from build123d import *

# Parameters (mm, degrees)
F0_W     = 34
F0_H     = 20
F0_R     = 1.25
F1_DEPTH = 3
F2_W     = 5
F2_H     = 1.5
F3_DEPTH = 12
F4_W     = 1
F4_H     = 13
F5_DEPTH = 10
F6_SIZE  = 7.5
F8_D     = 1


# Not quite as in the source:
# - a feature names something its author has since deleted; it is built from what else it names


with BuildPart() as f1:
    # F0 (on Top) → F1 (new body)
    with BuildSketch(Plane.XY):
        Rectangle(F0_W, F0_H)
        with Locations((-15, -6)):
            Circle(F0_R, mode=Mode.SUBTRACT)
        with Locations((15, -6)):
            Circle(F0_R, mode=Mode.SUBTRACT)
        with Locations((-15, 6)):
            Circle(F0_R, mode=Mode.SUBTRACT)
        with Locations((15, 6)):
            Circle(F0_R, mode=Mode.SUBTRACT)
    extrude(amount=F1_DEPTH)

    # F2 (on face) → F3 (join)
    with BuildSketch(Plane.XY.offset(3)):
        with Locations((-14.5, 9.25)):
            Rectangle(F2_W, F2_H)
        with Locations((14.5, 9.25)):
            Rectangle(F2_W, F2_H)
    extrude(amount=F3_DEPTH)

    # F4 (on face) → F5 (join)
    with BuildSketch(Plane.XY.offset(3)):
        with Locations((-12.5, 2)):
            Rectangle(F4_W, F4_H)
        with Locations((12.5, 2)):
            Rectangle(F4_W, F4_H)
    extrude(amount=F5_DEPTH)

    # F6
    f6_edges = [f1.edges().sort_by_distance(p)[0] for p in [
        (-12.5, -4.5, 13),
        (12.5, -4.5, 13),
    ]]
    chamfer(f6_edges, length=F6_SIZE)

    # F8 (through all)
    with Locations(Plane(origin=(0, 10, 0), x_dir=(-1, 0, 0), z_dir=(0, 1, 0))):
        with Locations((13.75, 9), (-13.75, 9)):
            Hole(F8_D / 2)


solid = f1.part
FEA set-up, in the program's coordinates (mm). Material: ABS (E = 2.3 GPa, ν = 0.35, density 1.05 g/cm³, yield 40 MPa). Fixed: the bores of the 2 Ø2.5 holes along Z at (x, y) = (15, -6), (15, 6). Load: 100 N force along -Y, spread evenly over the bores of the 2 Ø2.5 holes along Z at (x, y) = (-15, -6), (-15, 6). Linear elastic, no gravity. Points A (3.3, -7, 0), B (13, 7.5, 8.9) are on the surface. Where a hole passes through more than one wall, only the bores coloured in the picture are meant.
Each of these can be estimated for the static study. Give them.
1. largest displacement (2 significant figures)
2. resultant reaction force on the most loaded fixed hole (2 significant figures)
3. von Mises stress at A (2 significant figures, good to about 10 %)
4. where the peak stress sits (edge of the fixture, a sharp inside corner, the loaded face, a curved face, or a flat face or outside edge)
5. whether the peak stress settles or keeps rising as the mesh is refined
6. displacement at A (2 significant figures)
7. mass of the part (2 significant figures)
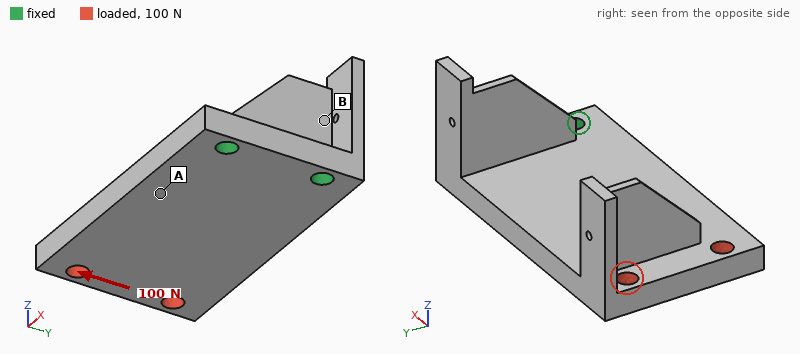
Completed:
0.34 mm
230 N
6.8 MPa
edge of the fixture
keeps rising
0.093 mm
2.5 g
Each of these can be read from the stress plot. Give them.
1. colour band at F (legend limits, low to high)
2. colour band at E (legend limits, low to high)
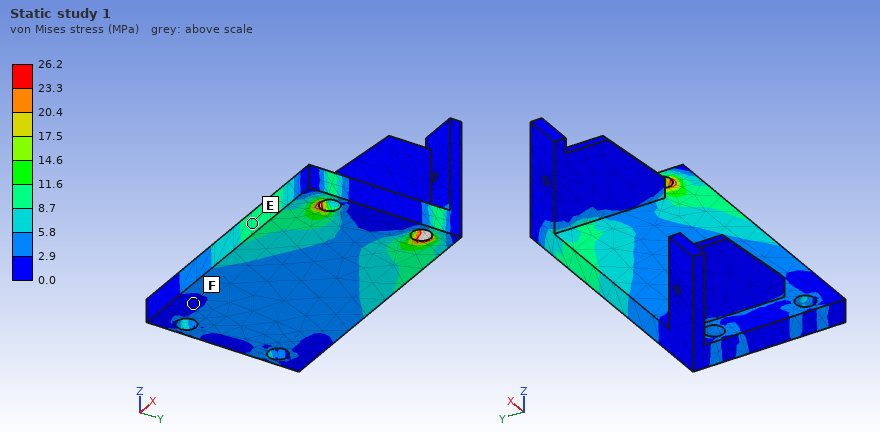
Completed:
0.0 to 2.9 MPa
8.7 to 11.6 MPa
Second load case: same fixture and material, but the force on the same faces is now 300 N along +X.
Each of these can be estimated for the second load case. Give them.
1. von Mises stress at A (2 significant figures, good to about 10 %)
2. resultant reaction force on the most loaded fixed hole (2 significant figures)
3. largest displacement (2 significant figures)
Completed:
5.1 MPa
150 N
99 µm
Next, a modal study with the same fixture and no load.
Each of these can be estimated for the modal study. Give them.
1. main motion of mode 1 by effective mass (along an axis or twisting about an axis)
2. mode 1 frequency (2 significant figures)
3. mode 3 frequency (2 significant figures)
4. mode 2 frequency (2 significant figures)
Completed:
along Z
630 Hz
2900 Hz
1800 Hz
